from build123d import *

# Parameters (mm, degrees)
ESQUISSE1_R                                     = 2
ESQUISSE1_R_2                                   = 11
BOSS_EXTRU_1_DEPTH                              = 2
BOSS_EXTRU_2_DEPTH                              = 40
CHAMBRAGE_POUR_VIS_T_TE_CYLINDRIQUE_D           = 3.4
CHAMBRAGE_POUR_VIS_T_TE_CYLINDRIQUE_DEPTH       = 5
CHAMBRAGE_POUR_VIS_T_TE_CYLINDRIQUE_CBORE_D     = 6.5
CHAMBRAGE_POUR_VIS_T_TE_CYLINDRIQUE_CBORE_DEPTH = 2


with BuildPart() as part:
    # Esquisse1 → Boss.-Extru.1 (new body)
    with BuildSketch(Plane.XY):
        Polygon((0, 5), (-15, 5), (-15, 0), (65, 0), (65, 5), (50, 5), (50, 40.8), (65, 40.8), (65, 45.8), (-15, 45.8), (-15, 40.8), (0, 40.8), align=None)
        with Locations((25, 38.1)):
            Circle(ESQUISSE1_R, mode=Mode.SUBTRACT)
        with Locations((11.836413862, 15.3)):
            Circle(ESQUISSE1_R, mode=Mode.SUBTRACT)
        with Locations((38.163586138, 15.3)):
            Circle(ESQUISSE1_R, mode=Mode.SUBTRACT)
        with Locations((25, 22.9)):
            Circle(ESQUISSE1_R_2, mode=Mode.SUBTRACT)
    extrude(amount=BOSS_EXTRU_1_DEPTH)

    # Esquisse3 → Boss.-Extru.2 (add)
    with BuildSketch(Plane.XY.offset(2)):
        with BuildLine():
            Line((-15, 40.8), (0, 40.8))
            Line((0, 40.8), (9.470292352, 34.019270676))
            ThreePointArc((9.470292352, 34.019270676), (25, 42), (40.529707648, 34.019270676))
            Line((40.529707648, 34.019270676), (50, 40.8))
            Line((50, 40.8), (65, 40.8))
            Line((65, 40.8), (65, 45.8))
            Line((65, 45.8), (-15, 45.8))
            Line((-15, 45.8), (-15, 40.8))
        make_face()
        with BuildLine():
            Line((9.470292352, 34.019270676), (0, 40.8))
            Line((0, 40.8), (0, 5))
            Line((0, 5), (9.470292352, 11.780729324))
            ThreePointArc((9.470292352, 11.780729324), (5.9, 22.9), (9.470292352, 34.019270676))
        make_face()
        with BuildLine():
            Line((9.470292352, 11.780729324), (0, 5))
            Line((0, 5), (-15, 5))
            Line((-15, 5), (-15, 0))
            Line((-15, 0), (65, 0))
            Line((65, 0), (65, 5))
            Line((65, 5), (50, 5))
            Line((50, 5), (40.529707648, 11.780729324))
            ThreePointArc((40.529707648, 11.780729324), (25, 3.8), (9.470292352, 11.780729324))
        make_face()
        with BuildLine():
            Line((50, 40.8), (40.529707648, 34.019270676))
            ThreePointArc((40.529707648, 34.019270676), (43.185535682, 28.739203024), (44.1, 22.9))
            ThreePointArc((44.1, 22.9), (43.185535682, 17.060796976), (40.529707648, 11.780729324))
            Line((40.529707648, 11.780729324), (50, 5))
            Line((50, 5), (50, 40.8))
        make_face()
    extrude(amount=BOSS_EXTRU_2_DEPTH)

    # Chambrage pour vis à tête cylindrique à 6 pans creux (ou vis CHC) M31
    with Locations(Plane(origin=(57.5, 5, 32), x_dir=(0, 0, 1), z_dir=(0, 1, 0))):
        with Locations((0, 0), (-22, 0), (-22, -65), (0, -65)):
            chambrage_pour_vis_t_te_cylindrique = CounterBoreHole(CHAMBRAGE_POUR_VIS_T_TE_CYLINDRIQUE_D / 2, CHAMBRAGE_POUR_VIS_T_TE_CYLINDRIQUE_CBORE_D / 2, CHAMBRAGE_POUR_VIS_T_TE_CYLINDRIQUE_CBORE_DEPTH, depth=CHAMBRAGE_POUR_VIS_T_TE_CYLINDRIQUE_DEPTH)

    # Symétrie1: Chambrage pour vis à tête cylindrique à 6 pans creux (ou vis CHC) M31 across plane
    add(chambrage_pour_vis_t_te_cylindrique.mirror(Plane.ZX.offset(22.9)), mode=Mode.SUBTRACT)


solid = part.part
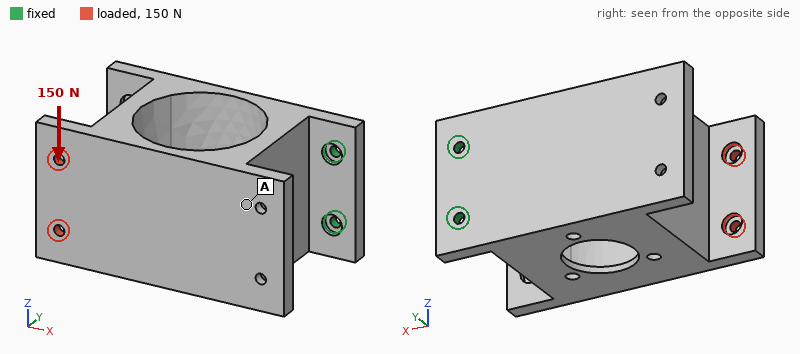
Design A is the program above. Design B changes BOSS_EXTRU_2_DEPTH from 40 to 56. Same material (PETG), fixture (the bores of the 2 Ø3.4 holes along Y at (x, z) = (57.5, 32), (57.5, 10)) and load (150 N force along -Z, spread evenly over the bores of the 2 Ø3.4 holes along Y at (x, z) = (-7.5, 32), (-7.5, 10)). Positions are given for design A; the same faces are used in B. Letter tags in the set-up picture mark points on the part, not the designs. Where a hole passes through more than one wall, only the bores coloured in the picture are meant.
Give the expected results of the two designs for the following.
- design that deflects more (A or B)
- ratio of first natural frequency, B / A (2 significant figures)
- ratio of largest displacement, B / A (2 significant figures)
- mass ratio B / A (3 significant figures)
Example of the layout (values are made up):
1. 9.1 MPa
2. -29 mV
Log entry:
1. A
2. 0.88
3. 0.87
4. 1.38
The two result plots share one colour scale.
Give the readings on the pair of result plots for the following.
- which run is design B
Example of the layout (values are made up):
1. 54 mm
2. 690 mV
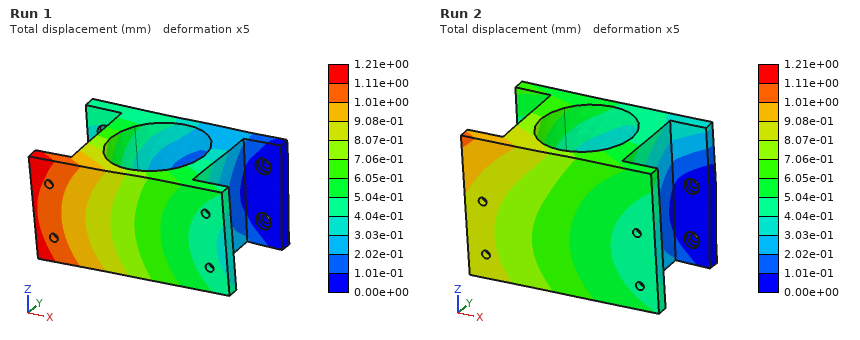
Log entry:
1. Run 2
